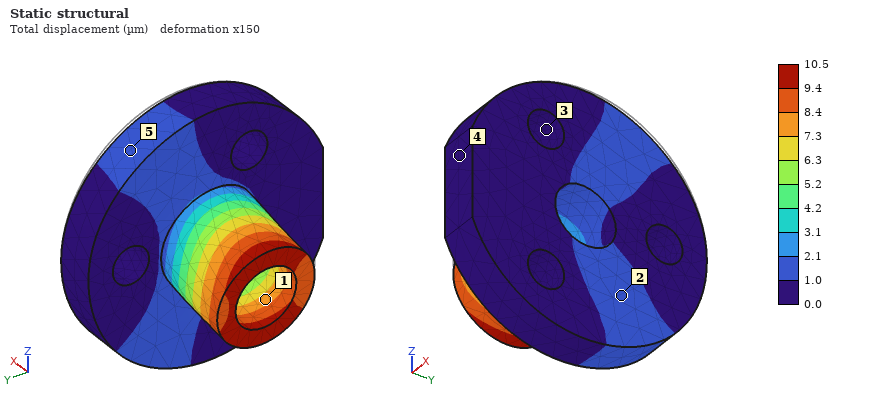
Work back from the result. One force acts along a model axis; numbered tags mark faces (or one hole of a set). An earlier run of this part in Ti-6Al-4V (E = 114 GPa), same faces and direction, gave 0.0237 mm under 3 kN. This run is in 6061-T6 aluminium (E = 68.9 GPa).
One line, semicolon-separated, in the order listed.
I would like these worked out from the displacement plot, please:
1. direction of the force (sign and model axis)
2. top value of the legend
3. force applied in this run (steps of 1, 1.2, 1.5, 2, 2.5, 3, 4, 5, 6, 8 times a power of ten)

-Z; 10.5 µm; 800 N
